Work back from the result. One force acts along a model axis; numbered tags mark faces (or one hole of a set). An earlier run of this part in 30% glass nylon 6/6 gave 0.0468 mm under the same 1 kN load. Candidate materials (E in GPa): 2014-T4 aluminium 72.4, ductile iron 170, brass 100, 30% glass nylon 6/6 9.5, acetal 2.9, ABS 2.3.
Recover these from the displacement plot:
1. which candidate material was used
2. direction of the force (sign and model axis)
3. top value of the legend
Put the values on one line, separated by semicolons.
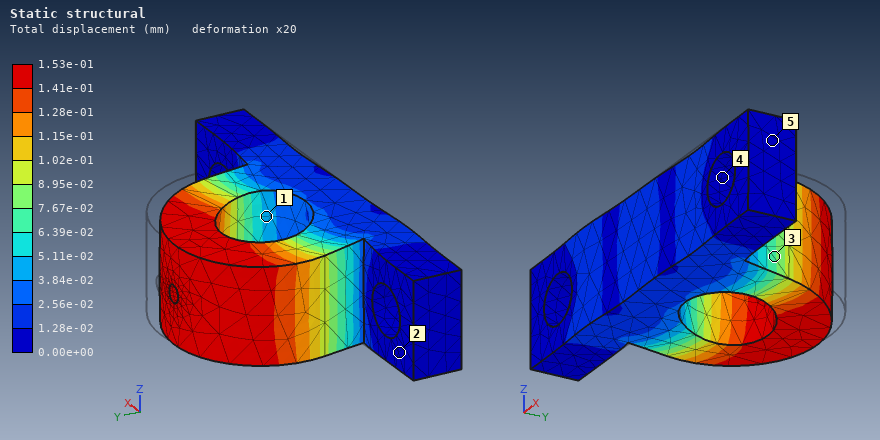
acetal; -X; 1.53e-01 mm
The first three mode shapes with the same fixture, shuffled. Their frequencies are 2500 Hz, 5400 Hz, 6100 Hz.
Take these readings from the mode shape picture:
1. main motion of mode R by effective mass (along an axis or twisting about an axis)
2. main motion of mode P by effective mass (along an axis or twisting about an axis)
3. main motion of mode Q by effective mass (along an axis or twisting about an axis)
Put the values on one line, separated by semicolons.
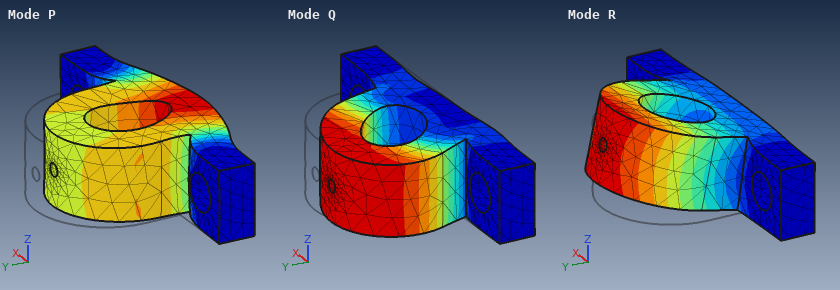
along Z; along Y; along X
